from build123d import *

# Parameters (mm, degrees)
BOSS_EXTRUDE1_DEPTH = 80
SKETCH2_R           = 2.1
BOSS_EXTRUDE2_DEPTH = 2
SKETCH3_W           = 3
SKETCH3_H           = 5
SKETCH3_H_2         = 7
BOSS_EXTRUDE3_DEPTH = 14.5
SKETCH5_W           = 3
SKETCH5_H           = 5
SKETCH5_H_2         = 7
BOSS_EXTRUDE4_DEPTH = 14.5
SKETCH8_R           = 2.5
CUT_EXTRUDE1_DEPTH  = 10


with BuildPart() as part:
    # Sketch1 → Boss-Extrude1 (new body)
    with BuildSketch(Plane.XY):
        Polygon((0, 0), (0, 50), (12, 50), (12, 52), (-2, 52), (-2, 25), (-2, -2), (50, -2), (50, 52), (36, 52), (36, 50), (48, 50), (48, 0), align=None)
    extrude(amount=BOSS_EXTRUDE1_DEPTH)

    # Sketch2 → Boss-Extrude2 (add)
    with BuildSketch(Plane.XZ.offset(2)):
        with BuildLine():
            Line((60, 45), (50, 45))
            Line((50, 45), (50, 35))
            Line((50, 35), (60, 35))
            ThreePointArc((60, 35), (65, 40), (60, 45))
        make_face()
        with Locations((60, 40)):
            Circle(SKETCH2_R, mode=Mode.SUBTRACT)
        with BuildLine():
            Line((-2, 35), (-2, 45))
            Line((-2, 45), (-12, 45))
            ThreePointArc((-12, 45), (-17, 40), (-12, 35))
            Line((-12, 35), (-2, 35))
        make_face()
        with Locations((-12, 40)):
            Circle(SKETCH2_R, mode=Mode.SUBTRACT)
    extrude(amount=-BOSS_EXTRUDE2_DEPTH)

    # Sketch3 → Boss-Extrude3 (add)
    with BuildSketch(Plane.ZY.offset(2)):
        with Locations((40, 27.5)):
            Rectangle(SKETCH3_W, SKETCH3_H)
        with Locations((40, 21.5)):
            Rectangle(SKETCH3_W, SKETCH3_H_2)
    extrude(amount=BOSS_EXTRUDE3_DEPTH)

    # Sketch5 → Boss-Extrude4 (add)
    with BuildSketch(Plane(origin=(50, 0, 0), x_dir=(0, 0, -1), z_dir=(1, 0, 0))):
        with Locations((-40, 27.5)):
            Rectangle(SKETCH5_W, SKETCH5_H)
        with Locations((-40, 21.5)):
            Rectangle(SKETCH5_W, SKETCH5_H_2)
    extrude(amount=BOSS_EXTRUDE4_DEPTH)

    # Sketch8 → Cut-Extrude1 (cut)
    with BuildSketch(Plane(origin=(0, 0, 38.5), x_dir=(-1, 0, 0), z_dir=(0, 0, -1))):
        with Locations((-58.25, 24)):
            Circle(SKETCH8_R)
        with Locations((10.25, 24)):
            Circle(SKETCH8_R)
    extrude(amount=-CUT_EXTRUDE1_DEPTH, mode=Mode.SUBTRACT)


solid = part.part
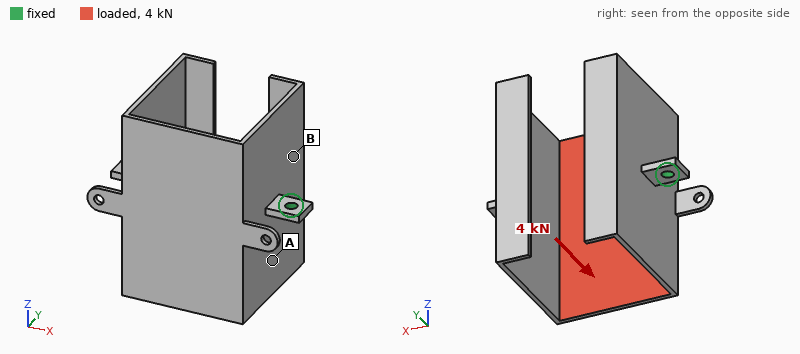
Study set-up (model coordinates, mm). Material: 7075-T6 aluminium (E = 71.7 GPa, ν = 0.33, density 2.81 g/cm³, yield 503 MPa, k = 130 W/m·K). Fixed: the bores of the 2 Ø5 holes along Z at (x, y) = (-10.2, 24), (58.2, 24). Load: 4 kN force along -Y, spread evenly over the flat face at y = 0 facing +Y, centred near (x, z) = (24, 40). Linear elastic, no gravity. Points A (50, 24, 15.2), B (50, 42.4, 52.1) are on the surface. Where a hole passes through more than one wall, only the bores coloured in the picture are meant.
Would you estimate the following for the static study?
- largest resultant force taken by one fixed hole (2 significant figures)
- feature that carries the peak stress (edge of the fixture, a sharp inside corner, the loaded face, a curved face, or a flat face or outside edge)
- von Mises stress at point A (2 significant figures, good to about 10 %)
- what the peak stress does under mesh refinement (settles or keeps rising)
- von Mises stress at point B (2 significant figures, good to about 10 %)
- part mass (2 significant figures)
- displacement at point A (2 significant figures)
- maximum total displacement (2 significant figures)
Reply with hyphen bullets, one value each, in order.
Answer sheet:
- 2.1 kN
- edge of the fixture
- 22 MPa
- keeps rising
- 41 MPa
- 85 g
- 0.20 mm
- 0.83 mm
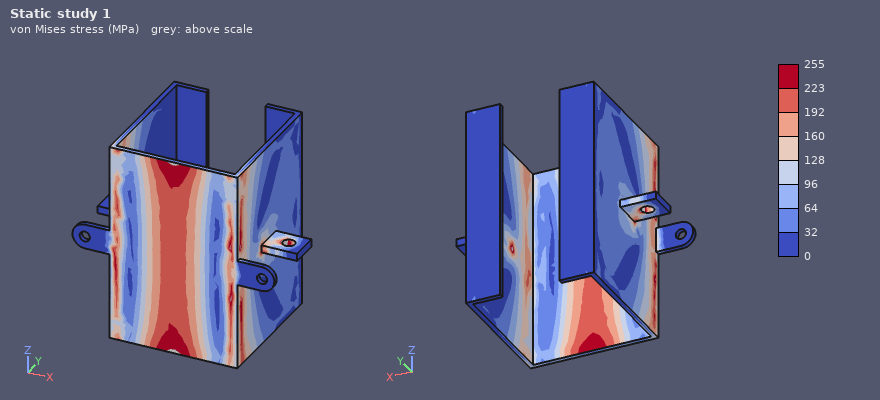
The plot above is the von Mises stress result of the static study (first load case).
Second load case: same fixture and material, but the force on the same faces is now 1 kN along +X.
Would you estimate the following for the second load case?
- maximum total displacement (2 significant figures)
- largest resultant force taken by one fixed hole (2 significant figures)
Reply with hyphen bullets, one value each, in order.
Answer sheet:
- 0.47 mm
- 540 N
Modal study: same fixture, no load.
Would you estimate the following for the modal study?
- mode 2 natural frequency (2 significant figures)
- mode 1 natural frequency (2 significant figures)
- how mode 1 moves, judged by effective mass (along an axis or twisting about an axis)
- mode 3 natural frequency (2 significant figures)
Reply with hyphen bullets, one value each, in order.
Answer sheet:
- 620 Hz
- 570 Hz
- twisting about X
- 810 Hz
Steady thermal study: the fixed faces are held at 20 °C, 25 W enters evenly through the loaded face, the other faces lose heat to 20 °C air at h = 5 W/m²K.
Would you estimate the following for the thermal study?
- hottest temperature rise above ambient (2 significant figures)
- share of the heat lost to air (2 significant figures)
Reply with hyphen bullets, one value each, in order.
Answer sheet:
- 46 K
- 16 %
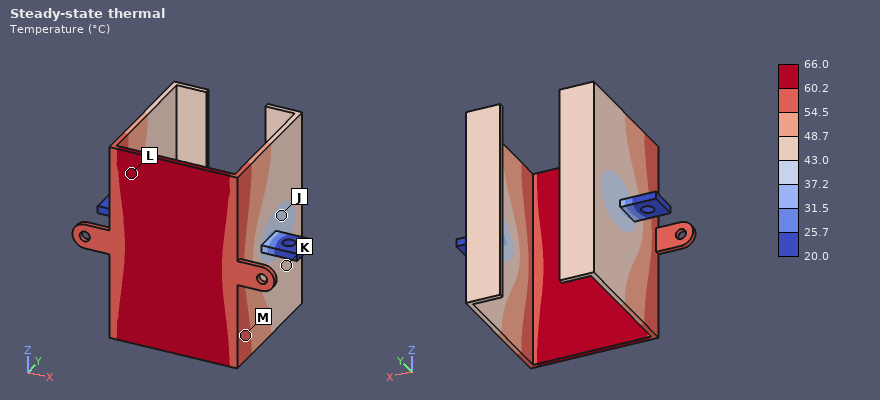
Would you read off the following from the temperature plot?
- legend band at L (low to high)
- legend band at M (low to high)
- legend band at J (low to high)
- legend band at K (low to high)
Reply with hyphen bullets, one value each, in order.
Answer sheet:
- 60.2 to 66.0 °C
- 54.5 to 60.2 °C
- 37.2 to 43.0 °C
- 43.0 to 48.7 °C
